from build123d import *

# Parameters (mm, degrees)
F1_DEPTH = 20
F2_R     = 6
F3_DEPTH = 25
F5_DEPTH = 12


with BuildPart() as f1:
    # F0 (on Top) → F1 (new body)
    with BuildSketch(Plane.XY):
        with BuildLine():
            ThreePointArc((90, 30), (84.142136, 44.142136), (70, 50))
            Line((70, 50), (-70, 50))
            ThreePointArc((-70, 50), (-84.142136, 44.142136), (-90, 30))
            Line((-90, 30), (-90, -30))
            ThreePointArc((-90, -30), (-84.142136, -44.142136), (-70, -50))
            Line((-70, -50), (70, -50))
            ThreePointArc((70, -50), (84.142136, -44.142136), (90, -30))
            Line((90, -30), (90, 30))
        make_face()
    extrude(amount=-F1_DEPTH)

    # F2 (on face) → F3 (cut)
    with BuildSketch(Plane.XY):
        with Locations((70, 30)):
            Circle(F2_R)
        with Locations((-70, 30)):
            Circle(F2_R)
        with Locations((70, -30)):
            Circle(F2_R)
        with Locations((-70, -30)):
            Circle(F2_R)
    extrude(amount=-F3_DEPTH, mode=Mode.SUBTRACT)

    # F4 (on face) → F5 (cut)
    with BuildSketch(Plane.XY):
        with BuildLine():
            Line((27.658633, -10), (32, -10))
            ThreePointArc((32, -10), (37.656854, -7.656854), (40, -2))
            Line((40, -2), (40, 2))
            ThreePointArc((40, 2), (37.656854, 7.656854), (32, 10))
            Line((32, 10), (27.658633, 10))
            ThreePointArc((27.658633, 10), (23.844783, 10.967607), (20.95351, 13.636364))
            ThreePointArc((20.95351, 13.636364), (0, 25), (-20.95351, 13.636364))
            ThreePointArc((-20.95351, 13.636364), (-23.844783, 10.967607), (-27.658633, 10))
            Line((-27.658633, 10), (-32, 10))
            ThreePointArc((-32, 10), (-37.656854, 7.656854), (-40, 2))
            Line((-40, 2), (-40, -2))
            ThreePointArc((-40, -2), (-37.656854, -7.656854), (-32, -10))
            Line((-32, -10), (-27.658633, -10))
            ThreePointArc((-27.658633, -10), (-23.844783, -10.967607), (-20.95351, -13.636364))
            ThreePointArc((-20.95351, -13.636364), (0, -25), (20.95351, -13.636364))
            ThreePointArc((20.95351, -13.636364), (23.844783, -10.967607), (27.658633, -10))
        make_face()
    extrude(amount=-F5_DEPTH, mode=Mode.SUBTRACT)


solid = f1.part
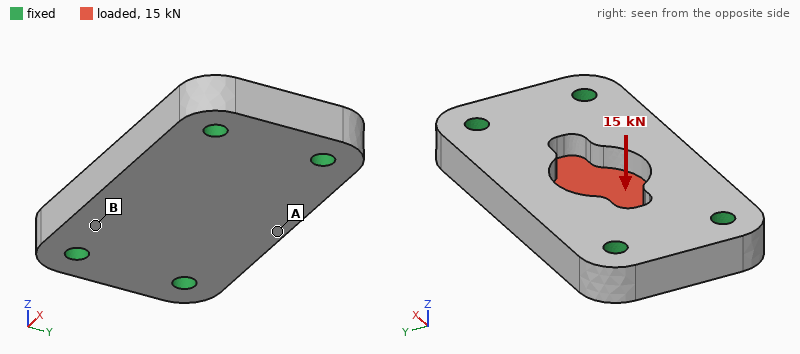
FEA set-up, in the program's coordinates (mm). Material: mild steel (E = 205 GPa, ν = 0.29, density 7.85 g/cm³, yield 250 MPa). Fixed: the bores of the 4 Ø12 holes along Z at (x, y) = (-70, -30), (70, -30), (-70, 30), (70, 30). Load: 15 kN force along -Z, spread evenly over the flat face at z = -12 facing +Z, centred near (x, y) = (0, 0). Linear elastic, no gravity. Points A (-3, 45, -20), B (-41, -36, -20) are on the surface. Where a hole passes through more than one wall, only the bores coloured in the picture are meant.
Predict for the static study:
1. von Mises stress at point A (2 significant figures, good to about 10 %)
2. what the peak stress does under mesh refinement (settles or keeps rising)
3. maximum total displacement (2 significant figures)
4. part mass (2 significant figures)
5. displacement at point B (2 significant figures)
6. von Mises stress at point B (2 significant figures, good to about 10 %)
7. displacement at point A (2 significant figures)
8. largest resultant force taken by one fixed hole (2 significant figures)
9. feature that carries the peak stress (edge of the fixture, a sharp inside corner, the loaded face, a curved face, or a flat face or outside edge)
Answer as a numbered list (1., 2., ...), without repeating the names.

1. 23 MPa
2. keeps rising
3. 33 µm
4. 2.5 kg
5. 7.5 µm
6. 8.7 MPa
7. 14 µm
8. 4.0 kN
9. edge of the fixture
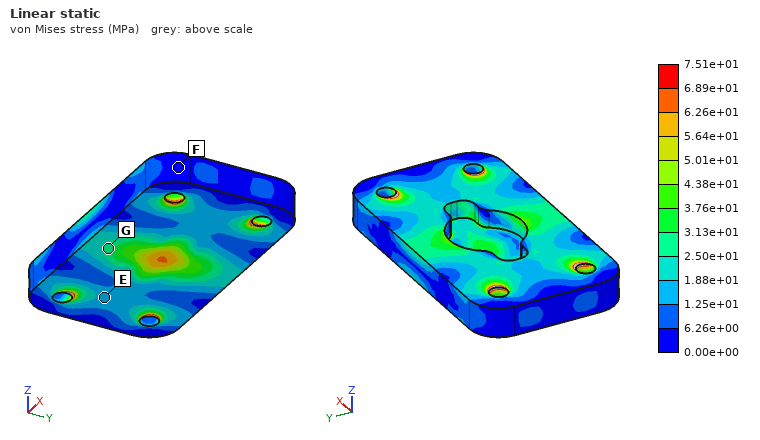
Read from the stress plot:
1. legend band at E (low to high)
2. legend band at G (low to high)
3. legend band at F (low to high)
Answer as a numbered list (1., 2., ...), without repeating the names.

1. 1.25e+01 to 1.88e+01 MPa
2. 2.50e+01 to 3.13e+01 MPa
3. 0.00e+00 to 6.26e+00 MPa
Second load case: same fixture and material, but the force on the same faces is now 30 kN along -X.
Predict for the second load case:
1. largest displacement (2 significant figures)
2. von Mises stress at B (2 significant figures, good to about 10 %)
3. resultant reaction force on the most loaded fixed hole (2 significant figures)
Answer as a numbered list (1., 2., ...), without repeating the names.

1. 6.7 µm
2. 8.4 MPa
3. 7.7 kN
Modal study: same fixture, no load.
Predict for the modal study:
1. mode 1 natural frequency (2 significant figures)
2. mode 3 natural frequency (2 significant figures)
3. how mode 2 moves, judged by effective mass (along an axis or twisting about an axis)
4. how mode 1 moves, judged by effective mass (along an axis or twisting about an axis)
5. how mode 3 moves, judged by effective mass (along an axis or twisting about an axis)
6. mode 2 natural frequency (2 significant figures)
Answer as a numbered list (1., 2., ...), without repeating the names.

1. 4900 Hz
2. 9900 Hz
3. twisting about X
4. along Z
5. along Y
6. 5900 Hz
